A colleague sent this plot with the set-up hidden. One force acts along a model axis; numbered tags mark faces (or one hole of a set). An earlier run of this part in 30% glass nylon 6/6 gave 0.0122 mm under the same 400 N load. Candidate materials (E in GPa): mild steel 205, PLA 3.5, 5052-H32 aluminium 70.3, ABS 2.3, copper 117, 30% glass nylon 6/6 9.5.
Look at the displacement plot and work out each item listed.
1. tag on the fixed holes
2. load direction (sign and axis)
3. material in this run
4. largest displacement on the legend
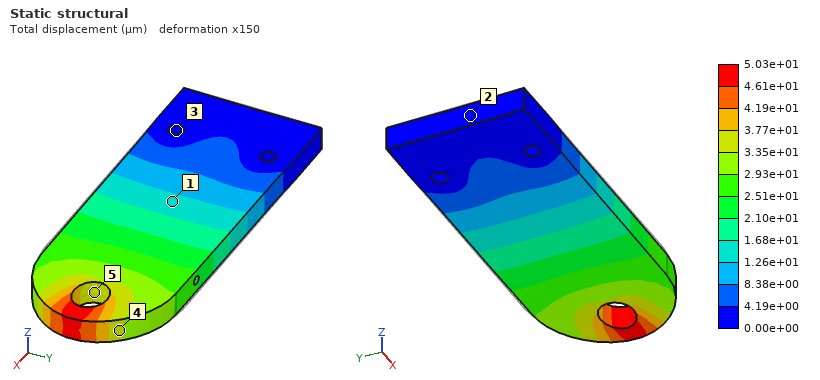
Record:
3
+X
ABS
5.03e+01 µm
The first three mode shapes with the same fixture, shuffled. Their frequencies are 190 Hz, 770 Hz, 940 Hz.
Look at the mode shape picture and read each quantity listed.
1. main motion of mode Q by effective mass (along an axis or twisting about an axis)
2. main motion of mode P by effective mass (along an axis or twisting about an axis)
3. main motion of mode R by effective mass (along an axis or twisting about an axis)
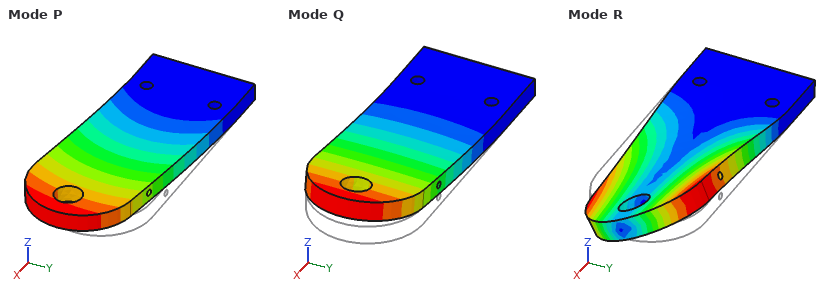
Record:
along Z
along Y
twisting about X
